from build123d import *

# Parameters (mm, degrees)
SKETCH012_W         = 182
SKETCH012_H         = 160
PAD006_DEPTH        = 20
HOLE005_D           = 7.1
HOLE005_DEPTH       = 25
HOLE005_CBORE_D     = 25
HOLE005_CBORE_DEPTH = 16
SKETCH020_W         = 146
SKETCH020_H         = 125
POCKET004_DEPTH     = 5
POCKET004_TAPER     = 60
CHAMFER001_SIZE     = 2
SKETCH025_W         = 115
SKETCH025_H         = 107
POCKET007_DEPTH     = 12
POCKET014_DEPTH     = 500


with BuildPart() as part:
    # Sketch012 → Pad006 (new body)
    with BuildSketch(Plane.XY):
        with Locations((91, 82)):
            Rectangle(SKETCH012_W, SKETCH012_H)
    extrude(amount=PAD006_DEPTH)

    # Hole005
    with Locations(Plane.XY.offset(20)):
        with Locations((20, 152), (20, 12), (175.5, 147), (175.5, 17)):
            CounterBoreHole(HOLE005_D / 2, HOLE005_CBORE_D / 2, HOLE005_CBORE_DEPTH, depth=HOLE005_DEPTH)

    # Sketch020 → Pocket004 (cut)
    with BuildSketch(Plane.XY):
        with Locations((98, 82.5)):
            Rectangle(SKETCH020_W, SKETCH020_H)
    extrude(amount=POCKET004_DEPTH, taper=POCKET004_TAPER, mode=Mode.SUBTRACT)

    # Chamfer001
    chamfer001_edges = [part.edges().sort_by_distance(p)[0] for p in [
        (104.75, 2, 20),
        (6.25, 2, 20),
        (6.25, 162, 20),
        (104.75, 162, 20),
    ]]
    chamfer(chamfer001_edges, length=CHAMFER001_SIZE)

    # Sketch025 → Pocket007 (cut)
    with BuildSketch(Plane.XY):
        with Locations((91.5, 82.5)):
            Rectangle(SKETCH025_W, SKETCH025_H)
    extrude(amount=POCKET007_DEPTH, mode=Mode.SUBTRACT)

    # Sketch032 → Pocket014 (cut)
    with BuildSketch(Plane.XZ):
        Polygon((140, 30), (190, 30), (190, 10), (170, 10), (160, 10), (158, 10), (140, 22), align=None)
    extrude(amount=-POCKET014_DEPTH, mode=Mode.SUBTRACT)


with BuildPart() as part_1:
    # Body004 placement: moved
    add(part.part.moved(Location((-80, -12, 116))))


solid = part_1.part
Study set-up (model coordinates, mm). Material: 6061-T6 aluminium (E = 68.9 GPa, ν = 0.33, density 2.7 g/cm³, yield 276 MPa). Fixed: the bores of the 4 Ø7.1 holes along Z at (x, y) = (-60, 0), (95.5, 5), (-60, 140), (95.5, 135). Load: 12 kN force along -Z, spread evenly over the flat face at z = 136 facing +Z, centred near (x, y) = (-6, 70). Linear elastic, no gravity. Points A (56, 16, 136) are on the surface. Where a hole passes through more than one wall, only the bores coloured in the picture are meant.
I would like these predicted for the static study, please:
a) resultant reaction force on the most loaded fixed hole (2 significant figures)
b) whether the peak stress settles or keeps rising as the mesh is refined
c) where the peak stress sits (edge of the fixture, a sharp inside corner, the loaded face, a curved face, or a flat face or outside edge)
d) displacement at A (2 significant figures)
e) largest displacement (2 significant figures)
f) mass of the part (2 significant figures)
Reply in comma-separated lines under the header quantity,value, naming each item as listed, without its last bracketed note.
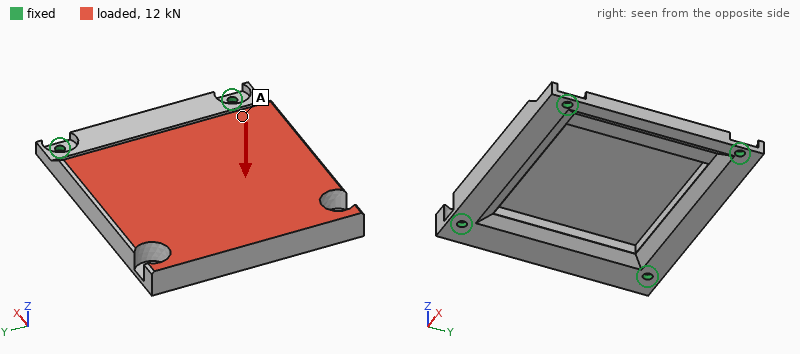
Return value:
quantity,value
resultant reaction force on the most loaded fixed hole,7.0 kN
whether the peak stress settles or keeps rising as the mesh is refined,keeps rising
where the peak stress sits,edge of the fixture
displacement at A,0.088 mm
largest displacement,0.19 mm
mass of the part,930 g
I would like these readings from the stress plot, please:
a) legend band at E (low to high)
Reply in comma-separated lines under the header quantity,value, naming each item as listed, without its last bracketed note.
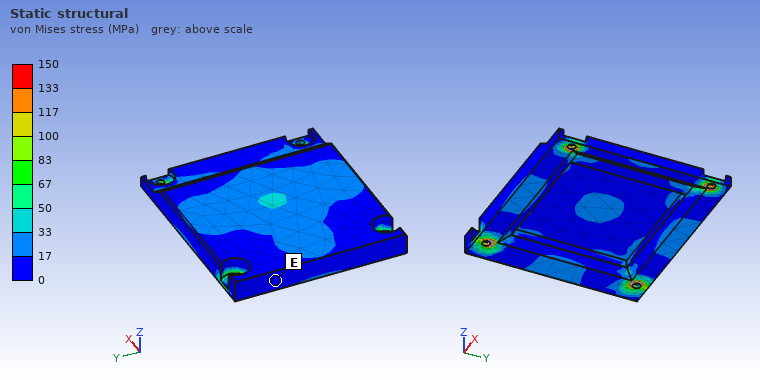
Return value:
quantity,value
legend band at E,0 to 17 MPa
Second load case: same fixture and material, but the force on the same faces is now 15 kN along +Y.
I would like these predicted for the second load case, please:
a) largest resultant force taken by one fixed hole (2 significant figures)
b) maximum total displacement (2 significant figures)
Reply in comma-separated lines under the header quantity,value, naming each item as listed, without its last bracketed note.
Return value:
quantity,value
largest resultant force taken by one fixed hole,5.1 kN
maximum total displacement,35 µm
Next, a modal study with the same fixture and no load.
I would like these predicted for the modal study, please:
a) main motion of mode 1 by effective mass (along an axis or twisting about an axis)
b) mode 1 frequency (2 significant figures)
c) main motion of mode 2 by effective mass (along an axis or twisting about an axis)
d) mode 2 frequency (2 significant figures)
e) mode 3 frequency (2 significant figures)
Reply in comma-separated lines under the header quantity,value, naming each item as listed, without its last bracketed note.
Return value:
quantity,value
main motion of mode 1 by effective mass,along Z
mode 1 frequency,1900 Hz
main motion of mode 2 by effective mass,twisting about X
mode 2 frequency,2500 Hz
mode 3 frequency,2600 Hz
